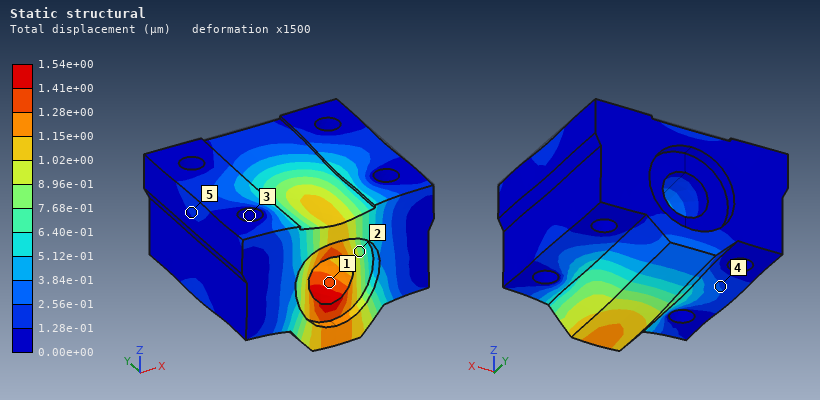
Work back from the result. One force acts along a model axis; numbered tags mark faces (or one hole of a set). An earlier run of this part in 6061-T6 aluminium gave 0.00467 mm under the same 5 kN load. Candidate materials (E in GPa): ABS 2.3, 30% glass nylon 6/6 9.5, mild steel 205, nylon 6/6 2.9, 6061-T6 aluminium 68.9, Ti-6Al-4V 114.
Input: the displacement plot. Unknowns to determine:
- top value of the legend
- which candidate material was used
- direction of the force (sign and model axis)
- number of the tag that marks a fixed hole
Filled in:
1.54e+00 µm
mild steel
-Z
3
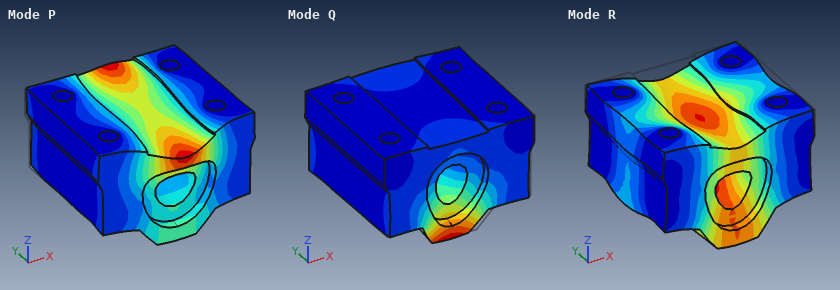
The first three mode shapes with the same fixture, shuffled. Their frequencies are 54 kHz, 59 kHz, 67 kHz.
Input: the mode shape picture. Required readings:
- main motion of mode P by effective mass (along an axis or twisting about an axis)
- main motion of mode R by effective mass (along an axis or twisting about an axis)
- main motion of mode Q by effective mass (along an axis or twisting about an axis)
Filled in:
along Y
along Z
along Y
